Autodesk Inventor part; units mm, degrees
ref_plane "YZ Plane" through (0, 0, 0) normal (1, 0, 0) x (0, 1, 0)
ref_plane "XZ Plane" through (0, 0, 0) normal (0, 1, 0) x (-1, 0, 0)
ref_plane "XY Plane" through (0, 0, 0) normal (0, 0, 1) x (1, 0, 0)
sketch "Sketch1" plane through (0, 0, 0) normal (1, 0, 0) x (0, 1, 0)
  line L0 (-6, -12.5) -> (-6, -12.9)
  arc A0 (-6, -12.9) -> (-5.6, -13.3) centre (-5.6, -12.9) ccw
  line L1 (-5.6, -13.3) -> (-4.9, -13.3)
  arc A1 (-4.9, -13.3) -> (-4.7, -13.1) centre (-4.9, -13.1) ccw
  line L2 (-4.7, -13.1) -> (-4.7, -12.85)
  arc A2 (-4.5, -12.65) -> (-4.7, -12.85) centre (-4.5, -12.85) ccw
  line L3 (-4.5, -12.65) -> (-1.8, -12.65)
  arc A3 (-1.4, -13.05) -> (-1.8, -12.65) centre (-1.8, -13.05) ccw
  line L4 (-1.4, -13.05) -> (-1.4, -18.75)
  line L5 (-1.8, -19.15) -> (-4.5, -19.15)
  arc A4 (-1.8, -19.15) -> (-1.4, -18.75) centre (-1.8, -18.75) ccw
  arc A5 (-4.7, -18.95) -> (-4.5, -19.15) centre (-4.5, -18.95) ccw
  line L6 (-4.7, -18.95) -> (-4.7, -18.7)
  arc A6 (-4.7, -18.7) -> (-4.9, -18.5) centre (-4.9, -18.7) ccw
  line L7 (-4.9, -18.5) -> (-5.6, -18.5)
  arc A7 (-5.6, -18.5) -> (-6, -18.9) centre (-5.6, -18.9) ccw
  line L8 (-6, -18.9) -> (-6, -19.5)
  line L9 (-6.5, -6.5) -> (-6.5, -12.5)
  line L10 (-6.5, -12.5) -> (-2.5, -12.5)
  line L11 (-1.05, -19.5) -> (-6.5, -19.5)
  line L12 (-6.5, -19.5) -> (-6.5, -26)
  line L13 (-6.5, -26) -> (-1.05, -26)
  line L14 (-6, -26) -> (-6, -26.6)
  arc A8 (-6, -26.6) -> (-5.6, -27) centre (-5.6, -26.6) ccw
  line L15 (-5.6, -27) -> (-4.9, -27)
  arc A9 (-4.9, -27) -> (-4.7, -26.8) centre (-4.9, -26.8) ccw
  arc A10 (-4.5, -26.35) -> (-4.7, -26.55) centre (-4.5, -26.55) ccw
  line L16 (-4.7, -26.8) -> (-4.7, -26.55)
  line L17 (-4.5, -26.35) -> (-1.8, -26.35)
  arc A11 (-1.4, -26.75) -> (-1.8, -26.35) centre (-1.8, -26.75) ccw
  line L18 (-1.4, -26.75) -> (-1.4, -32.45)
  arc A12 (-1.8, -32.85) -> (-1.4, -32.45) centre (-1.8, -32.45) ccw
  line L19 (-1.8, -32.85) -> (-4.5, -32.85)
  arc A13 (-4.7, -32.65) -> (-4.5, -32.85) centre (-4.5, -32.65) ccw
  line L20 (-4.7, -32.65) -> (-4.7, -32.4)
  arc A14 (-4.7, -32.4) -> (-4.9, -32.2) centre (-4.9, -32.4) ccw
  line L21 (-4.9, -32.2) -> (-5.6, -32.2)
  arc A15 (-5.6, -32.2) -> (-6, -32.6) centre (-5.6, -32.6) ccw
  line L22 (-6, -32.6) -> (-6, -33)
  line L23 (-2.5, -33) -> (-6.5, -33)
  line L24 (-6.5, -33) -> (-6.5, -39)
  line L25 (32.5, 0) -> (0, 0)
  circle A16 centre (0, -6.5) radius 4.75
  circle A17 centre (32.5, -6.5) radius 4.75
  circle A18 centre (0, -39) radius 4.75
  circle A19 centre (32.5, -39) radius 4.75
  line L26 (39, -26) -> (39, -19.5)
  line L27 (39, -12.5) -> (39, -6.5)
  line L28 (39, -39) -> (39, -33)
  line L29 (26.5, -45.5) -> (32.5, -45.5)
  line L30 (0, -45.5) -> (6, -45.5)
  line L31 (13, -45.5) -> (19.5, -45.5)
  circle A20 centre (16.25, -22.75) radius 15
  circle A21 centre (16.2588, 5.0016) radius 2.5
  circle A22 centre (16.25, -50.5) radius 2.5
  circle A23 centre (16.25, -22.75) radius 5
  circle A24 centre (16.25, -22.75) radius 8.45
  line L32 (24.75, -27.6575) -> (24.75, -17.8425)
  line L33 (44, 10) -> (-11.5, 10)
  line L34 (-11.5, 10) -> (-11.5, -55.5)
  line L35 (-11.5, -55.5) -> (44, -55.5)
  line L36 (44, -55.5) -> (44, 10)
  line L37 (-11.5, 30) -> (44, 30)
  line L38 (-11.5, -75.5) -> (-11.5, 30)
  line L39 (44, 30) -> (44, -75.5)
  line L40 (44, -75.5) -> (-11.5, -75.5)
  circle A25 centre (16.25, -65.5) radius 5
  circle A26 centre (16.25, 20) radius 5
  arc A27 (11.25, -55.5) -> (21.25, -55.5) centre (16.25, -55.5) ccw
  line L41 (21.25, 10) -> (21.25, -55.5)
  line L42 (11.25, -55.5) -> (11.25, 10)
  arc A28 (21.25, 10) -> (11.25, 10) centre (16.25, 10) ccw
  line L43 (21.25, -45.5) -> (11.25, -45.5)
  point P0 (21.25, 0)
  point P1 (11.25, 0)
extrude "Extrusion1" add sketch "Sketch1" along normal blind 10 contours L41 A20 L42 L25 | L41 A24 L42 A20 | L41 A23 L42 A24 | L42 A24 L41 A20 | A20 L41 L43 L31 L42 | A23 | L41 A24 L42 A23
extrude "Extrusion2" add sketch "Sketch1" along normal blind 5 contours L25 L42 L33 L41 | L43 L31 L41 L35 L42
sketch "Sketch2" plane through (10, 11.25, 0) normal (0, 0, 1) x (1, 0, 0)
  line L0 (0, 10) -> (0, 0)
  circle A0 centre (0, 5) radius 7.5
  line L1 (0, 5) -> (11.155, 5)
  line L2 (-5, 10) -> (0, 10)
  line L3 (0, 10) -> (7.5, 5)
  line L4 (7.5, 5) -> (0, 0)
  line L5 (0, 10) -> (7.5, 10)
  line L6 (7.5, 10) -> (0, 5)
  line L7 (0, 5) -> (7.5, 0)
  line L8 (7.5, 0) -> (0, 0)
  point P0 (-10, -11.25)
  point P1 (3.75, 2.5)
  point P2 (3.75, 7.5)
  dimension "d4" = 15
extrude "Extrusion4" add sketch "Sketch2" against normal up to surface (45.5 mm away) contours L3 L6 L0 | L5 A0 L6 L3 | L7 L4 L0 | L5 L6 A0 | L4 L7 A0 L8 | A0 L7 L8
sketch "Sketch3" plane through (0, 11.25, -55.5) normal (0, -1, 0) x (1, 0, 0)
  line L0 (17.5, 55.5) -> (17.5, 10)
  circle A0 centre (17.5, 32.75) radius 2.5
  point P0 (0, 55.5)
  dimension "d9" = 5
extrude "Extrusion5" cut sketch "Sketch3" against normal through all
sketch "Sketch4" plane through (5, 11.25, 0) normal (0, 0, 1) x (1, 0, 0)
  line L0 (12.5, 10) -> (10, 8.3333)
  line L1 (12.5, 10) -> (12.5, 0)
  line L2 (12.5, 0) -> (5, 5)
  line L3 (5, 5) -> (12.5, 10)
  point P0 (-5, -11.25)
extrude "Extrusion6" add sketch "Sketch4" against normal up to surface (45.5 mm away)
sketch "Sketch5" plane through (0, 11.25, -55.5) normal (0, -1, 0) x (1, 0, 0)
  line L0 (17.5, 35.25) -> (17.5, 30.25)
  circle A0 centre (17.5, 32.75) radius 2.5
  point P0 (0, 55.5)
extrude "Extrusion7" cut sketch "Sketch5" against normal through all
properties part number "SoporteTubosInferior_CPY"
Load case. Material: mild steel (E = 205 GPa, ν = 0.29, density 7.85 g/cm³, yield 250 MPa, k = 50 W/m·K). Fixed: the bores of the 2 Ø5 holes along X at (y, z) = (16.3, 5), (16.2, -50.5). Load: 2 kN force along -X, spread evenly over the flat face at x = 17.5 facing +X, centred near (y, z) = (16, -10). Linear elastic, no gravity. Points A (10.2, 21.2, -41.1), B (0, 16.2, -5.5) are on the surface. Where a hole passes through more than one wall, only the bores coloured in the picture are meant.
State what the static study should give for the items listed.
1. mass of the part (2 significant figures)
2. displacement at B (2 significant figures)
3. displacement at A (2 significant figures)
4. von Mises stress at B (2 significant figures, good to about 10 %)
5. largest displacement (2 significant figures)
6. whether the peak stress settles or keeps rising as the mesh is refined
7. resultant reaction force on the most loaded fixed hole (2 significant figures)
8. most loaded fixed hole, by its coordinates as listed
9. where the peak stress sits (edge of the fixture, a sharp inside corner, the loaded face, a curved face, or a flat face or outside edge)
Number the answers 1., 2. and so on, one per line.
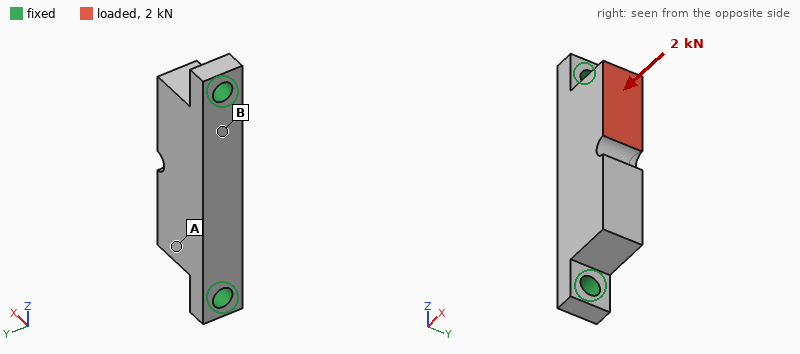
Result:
1. 68 g
2. 4.4 µm
3. 1.8 µm
4. 22 MPa
5. 5.5 µm
6. keeps rising
7. 1.7 kN
8. (16.3, 5)
9. edge of the fixture
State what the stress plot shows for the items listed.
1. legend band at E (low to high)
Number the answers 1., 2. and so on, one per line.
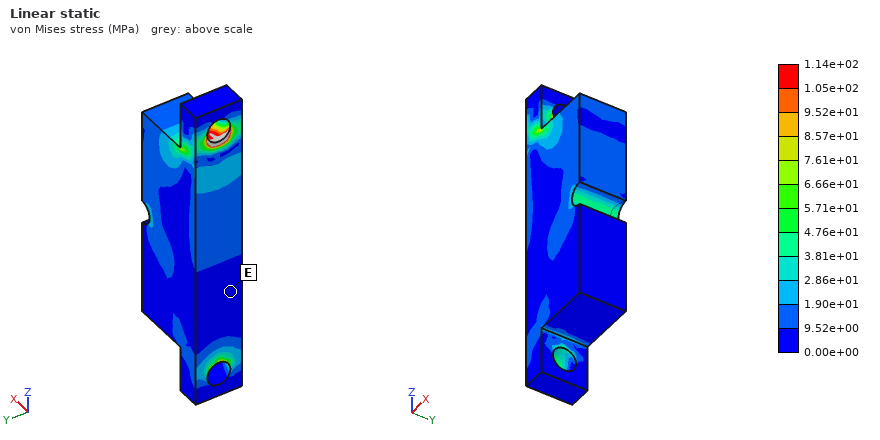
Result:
1. 0.00e+00 to 9.52e+00 MPa
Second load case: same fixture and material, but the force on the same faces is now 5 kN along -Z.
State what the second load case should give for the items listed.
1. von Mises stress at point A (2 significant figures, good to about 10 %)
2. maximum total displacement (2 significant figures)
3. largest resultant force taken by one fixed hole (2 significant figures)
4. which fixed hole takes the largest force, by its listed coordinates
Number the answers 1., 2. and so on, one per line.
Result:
1. 25 MPa
2. 13 µm
3. 3.3 kN
4. (16.2, -50.5)
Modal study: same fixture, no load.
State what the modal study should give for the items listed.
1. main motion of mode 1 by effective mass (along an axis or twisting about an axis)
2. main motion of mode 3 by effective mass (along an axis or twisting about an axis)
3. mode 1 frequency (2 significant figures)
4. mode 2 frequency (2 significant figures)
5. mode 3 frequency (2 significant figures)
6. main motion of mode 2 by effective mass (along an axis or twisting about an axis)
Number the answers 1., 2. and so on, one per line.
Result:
1. along Y
2. along Y
3. 6700 Hz
4. 14 kHz
5. 15 kHz
6. along X
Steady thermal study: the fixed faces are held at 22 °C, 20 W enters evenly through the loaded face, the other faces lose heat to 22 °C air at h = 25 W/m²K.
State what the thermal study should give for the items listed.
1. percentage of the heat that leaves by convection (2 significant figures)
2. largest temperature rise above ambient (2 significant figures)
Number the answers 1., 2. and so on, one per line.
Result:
1. 10 %
2. 55 K
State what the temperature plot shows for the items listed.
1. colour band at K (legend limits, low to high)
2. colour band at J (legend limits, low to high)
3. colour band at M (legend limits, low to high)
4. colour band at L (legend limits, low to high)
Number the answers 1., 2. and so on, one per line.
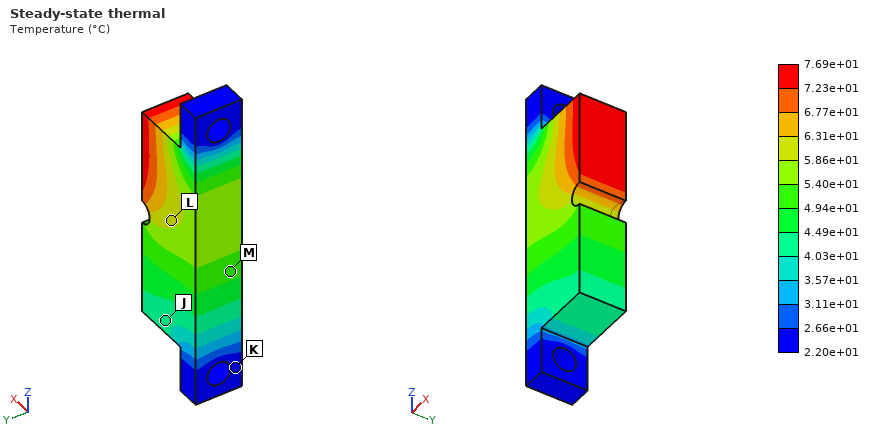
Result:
1. 2.20e+01 to 2.66e+01 °C
2. 4.03e+01 to 4.49e+01 °C
3. 4.94e+01 to 5.40e+01 °C
4. 5.86e+01 to 6.31e+01 °C
